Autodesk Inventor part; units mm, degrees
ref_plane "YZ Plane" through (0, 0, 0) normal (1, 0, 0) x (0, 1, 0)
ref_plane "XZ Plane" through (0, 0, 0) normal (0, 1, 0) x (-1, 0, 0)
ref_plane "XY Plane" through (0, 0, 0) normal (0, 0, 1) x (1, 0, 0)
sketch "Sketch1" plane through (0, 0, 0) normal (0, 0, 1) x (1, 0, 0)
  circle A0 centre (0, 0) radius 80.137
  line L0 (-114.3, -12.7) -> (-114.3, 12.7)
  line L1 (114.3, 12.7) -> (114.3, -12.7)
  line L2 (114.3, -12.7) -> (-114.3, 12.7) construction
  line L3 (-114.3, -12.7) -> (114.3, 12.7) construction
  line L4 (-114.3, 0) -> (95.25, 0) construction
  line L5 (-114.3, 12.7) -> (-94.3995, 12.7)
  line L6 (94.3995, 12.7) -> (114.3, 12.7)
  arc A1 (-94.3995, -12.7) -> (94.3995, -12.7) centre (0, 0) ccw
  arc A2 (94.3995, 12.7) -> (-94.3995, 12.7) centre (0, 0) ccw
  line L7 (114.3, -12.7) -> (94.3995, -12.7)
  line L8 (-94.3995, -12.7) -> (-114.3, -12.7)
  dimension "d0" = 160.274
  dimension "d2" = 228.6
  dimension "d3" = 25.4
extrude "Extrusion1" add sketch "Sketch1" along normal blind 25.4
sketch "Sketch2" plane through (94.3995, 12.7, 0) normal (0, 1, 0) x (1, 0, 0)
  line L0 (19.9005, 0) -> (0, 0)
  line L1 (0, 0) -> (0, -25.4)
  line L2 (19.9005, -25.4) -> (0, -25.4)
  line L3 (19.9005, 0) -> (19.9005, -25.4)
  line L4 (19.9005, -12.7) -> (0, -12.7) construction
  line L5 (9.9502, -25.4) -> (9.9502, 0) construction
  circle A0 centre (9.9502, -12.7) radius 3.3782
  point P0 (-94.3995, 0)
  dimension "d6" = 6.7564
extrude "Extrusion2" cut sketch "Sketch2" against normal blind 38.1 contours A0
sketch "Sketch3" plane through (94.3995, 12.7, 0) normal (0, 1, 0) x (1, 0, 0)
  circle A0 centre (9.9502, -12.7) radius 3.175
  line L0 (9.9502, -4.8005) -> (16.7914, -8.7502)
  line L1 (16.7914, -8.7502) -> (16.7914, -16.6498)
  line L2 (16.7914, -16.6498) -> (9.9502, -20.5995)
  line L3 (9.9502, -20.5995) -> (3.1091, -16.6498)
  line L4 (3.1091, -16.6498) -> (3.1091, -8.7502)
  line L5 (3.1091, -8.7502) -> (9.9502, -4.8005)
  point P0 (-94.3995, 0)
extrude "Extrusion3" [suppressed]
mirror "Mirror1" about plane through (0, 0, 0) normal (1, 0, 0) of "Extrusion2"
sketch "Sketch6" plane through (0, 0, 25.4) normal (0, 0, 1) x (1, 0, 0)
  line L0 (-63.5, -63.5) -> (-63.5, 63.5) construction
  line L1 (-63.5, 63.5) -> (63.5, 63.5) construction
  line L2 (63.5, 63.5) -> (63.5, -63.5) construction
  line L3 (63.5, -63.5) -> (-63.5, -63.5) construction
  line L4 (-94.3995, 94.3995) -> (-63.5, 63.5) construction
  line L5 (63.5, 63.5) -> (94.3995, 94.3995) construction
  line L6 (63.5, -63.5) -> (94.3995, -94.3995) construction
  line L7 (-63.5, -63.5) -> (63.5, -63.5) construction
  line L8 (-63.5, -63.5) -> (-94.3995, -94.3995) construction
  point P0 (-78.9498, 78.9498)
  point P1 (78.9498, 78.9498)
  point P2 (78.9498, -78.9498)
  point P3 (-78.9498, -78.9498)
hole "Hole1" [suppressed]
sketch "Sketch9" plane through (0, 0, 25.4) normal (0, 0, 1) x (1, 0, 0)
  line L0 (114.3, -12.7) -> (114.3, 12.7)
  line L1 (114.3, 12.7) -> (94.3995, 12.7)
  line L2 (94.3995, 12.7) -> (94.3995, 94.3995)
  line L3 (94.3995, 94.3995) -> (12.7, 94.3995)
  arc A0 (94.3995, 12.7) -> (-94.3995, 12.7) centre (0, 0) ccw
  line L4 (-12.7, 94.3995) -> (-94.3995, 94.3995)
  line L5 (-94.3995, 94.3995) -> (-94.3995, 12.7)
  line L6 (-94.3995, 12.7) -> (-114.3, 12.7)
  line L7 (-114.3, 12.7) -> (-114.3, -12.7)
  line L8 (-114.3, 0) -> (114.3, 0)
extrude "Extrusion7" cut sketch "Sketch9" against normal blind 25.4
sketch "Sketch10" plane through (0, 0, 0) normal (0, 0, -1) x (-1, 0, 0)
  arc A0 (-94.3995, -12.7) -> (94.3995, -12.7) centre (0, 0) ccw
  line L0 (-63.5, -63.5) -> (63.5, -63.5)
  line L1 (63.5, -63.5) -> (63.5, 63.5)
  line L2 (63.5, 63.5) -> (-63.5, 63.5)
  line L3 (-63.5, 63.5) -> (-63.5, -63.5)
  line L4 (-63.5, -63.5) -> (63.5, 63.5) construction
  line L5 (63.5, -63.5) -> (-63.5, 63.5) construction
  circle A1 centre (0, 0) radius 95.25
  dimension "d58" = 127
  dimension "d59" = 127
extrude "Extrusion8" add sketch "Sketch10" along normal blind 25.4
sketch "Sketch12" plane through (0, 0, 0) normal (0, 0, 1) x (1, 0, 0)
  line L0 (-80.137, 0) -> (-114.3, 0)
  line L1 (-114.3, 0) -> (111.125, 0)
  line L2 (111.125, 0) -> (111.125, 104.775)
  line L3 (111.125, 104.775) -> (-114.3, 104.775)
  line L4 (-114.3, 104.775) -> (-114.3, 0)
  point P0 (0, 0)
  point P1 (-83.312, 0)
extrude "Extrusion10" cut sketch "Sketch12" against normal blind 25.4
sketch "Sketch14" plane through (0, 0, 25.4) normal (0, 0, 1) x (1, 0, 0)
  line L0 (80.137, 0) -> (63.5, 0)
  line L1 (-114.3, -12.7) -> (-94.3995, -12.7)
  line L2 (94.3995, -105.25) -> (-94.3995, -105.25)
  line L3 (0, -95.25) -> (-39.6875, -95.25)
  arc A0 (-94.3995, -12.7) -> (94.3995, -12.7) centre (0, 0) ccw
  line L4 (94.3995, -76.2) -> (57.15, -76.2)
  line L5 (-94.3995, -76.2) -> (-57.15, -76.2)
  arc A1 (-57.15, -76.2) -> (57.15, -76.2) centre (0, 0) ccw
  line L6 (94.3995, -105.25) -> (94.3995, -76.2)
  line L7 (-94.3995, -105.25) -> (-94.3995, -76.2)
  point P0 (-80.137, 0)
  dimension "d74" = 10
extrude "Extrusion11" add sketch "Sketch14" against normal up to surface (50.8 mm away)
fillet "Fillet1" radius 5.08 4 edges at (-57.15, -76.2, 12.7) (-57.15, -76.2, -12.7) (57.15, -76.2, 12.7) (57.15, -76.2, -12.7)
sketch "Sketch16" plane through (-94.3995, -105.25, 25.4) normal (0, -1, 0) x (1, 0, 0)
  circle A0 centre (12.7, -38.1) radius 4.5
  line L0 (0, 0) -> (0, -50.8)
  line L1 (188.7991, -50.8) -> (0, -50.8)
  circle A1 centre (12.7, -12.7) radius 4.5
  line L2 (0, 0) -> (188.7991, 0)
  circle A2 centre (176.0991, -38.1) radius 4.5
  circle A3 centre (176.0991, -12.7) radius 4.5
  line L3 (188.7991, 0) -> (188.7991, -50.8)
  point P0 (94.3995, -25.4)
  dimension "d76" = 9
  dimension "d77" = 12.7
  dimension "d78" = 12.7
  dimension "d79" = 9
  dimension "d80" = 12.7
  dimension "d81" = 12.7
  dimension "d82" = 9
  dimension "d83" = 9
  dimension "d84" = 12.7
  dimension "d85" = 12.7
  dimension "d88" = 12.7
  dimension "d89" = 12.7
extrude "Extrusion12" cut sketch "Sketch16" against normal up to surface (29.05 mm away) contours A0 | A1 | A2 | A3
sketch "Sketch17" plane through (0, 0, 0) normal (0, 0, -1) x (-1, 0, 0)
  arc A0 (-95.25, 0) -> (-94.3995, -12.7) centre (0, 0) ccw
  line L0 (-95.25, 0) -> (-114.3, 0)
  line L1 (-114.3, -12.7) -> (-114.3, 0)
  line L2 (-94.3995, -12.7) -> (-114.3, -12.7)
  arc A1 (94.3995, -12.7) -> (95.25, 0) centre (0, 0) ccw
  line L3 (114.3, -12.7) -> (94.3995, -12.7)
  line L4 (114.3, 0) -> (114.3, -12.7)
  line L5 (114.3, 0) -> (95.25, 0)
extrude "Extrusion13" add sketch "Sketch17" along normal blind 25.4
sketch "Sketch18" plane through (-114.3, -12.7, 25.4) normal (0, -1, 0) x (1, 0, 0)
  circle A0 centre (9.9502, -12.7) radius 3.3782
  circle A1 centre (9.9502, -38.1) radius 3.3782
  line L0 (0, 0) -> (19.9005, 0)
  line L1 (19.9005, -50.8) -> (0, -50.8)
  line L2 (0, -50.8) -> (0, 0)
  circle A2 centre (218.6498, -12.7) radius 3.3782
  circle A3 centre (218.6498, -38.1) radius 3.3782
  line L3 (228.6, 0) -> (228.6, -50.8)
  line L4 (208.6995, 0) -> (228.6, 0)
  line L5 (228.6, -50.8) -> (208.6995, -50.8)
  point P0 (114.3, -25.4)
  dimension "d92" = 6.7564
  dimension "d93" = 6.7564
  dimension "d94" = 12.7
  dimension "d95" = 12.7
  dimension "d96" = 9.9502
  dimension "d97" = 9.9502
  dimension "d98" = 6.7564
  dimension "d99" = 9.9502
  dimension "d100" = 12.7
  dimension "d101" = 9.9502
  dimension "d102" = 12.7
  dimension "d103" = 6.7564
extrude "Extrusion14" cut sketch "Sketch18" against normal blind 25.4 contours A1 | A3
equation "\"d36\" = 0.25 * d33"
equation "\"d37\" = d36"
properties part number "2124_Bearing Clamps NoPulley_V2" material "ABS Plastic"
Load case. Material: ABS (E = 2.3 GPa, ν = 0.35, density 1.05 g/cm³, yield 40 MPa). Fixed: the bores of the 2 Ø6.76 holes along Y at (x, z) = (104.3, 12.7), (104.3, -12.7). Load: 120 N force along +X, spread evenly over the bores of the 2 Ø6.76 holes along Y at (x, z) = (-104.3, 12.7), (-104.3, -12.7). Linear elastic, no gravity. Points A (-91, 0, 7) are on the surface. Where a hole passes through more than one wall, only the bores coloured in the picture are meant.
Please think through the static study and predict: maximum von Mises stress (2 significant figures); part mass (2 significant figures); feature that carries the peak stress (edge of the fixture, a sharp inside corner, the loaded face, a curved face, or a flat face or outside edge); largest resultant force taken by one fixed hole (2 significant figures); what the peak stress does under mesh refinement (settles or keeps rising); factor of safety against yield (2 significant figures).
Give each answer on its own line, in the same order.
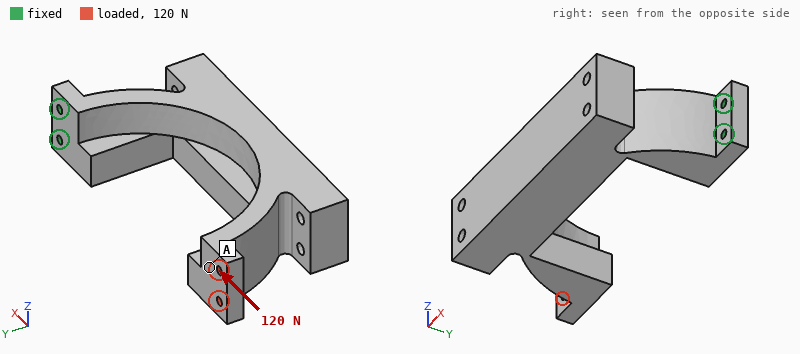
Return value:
7.8 MPa
510 g
a curved face
60 N
settles
5.1
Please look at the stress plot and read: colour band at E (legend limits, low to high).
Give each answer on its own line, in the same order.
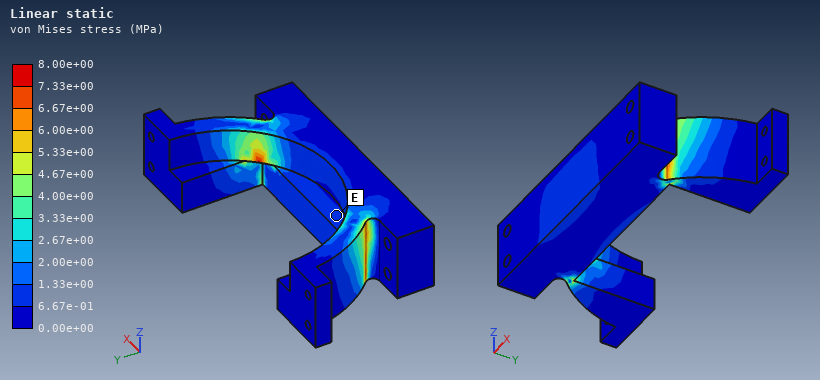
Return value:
6.67e-01 to 1.33e+00 MPa
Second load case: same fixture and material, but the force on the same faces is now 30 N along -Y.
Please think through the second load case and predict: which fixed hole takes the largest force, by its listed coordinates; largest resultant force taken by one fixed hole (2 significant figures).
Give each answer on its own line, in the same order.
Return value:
(104.3, 12.7)
22 N
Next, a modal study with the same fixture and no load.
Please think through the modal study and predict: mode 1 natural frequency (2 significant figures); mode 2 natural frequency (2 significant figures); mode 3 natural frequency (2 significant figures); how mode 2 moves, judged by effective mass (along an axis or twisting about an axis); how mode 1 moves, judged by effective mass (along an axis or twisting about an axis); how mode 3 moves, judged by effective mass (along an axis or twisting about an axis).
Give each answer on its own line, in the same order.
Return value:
39 Hz
71 Hz
180 Hz
along Z
along Y
along X
